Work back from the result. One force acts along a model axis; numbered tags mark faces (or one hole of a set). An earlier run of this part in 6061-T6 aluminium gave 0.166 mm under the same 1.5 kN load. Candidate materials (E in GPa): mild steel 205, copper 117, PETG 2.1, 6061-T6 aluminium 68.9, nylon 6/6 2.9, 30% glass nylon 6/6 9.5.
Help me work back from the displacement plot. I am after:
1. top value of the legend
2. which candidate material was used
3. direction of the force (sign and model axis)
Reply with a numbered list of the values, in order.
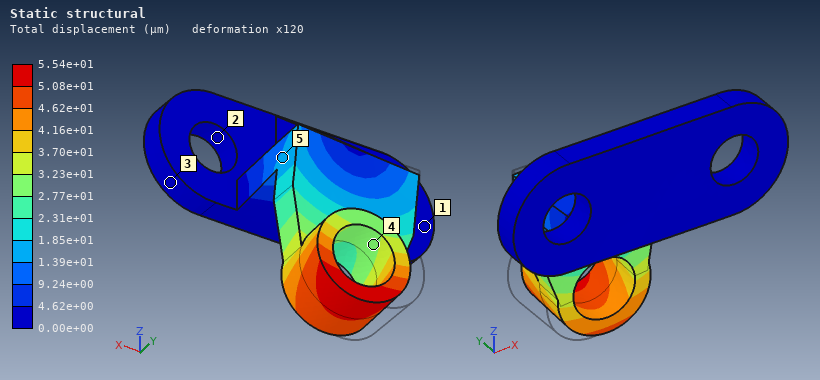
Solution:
1. 5.54e+01 µm
2. mild steel
3. +X
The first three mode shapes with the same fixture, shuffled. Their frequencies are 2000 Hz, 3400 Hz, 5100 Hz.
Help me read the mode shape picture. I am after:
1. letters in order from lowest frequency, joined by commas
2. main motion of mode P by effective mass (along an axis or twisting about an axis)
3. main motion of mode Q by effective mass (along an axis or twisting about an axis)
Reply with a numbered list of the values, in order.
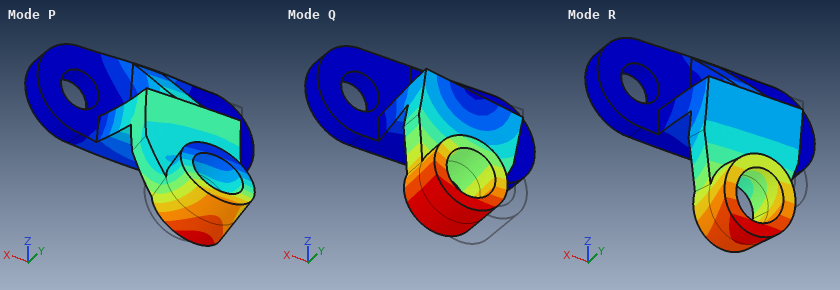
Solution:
1. R, Q, P
2. along Z
3. along X
